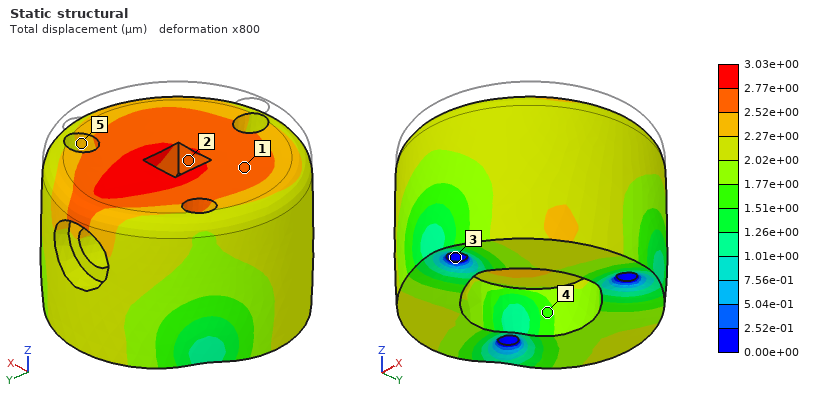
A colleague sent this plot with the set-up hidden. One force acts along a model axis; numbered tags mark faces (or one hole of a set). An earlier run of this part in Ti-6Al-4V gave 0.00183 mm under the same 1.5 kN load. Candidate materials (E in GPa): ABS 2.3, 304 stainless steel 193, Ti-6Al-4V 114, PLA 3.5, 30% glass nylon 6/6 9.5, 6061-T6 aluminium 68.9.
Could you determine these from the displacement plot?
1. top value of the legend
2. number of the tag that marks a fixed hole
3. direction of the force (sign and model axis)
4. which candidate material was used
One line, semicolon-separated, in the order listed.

3.03e+00 µm; 3; -Z; 6061-T6 aluminium
